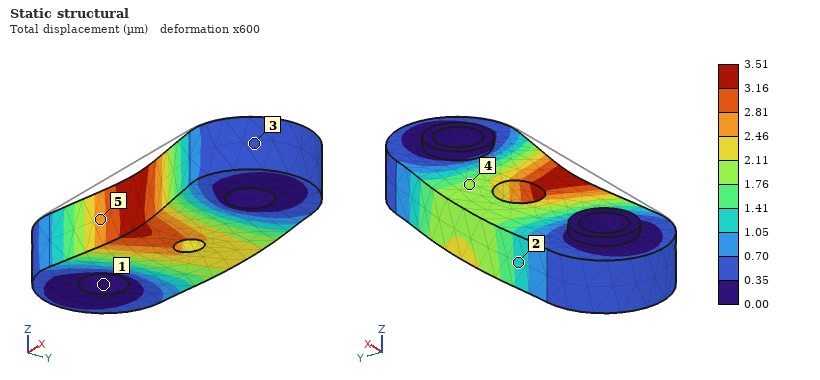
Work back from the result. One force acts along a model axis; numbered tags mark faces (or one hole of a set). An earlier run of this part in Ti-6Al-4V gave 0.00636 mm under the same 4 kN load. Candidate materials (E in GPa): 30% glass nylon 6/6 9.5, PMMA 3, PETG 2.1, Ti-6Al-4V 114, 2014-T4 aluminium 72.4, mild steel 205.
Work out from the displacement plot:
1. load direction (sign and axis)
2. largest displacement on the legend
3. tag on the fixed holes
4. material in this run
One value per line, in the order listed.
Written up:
+Y
3.51 µm
1
mild steel
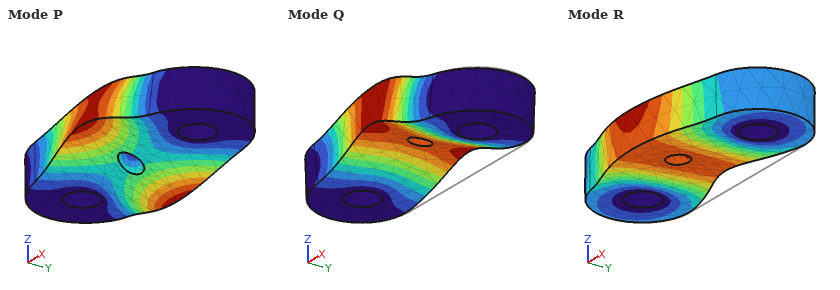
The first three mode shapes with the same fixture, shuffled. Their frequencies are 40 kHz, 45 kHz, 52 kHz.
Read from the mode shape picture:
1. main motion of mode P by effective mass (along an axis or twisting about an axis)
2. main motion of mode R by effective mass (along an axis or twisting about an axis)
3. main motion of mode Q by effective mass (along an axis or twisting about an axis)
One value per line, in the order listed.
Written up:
twisting about X
along Y
along Z
